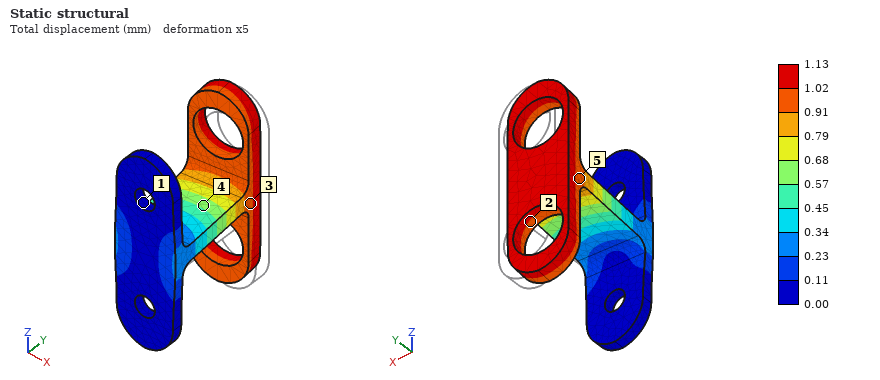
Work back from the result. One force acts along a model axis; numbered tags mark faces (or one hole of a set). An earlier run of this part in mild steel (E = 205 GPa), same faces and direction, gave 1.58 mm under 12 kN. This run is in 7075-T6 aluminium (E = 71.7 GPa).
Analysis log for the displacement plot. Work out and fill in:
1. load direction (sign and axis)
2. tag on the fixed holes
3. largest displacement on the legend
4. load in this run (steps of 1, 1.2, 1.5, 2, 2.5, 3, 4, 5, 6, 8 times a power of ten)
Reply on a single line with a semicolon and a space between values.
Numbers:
-X; 1; 1.13 mm; 3 kN
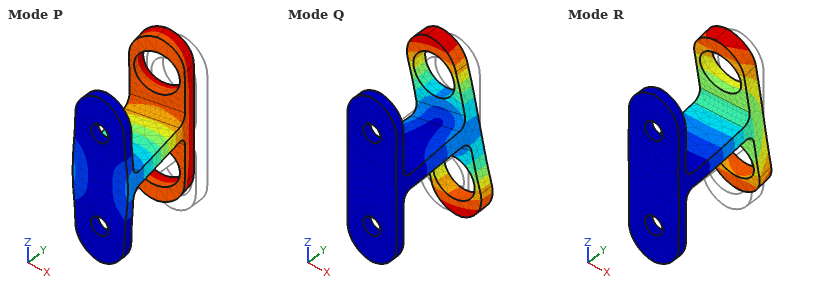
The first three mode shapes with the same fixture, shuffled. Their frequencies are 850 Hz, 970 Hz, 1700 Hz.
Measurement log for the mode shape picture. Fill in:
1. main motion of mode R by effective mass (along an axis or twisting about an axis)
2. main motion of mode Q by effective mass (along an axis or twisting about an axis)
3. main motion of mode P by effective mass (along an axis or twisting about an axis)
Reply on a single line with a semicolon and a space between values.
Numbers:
along Z; twisting about Y; along X
